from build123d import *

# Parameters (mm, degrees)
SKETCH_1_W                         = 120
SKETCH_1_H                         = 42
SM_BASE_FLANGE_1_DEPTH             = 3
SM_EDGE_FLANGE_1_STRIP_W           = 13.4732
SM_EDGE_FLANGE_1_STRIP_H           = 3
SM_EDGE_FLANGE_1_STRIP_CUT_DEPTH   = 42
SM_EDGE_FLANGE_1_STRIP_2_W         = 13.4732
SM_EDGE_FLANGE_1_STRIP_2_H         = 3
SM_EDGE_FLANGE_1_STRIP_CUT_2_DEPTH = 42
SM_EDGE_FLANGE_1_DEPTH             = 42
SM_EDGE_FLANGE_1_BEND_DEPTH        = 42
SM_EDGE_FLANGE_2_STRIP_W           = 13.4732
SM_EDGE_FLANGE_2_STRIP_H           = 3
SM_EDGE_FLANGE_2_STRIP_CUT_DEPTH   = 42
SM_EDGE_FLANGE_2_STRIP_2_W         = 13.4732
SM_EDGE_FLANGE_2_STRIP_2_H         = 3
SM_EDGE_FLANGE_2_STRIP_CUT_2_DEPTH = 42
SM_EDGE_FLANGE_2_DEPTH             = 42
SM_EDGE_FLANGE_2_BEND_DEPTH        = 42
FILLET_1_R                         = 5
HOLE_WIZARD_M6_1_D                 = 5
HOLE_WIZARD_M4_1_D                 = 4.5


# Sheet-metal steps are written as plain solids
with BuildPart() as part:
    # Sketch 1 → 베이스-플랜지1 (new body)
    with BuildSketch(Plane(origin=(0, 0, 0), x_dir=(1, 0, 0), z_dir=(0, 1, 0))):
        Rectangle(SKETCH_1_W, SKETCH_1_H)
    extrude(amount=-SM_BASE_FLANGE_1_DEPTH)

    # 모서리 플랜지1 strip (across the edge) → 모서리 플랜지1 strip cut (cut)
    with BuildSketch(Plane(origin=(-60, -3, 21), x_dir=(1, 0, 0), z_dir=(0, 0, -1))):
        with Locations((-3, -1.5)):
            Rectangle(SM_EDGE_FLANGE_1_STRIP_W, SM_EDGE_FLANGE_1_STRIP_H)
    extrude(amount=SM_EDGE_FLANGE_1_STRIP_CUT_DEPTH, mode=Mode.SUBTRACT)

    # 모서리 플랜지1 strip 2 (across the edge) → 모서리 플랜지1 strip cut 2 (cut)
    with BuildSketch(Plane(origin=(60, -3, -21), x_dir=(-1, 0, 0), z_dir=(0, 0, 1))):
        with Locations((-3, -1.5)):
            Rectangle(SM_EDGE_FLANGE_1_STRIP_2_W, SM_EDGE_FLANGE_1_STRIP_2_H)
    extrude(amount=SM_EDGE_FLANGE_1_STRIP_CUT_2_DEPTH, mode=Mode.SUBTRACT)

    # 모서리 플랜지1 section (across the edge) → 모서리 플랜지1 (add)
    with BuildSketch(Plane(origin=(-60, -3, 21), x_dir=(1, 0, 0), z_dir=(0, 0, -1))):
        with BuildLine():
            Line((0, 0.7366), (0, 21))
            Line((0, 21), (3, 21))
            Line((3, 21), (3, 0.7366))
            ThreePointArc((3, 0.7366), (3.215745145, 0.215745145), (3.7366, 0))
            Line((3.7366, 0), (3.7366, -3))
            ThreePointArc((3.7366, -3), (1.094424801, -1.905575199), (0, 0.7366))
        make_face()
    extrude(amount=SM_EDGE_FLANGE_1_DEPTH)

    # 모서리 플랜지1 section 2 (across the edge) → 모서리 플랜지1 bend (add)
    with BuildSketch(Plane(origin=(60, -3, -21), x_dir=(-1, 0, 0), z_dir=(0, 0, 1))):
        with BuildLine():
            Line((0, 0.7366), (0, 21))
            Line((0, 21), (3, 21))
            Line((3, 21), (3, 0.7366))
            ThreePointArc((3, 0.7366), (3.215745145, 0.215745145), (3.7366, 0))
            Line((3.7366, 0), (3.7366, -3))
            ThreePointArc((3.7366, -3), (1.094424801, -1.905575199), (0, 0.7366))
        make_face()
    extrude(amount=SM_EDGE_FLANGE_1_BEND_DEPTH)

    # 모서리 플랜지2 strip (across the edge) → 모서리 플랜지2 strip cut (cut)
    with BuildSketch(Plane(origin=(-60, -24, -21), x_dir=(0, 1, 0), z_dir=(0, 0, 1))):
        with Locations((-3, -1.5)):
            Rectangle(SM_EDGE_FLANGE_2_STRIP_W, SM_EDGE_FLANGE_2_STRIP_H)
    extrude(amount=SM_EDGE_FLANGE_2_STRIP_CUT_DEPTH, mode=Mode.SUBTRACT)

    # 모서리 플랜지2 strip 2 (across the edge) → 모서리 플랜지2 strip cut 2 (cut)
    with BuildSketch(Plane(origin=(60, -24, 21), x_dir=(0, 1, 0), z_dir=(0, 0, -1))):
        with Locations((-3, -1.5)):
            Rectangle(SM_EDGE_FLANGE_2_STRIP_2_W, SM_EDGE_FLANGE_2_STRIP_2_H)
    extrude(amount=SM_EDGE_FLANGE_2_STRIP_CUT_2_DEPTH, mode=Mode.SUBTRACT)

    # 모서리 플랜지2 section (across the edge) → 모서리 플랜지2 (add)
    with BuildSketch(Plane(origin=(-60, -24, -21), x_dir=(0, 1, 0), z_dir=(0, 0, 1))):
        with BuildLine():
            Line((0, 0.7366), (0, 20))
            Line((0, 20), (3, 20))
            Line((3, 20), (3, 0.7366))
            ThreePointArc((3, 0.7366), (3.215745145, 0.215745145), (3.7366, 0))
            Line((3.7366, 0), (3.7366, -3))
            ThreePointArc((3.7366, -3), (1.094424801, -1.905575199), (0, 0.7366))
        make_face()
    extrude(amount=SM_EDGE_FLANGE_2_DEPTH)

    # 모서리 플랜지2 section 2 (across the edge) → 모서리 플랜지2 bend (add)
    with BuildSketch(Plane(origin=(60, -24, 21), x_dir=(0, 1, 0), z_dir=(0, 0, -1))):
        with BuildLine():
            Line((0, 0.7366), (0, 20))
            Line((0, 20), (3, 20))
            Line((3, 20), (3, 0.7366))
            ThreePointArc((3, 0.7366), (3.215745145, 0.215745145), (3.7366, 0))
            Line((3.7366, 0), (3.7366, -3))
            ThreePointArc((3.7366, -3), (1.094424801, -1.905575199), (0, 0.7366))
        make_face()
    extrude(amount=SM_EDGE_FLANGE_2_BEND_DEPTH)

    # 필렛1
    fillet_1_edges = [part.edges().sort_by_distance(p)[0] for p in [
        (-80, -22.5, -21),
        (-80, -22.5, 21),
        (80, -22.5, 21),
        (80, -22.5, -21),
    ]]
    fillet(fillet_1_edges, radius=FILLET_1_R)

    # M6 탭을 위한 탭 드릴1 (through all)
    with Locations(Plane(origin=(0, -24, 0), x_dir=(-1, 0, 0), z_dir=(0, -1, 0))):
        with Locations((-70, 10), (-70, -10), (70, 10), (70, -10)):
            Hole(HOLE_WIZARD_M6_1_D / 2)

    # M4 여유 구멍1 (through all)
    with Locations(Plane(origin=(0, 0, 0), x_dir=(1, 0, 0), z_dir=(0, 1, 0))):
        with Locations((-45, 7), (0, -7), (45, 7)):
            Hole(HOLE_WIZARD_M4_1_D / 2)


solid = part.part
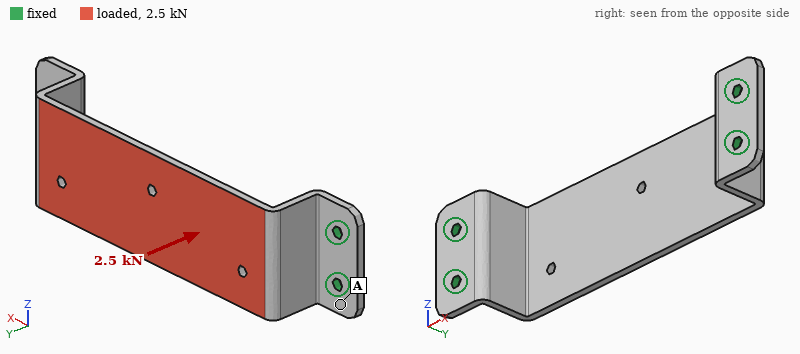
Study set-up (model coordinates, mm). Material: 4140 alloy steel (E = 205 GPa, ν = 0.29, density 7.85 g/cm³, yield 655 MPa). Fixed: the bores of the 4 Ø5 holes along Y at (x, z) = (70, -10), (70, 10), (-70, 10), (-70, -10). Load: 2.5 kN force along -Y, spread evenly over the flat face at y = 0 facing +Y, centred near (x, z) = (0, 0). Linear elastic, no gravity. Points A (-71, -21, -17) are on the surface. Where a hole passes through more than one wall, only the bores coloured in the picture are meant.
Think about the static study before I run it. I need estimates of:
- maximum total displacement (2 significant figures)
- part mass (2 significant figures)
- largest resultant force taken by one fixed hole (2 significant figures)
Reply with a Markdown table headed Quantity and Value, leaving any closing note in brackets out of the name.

| Quantity | Value |
|---|---|
| maximum total displacement | 0.74 mm |
| part mass | 190 g |
| largest resultant force taken by one fixed hole | 1.0 kN |
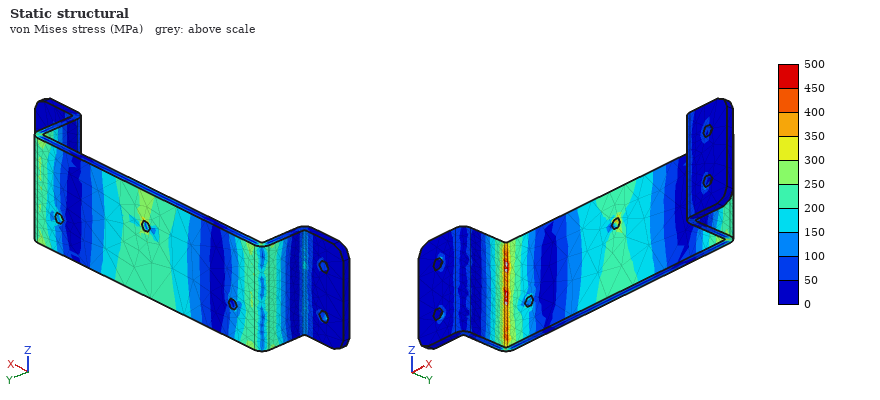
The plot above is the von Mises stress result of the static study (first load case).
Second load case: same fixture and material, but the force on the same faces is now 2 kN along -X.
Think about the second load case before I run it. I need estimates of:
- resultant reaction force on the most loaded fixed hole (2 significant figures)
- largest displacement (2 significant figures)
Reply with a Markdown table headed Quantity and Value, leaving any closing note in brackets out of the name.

| Quantity | Value |
|---|---|
| resultant reaction force on the most loaded fixed hole | 520 N |
| largest displacement | 0.21 mm |
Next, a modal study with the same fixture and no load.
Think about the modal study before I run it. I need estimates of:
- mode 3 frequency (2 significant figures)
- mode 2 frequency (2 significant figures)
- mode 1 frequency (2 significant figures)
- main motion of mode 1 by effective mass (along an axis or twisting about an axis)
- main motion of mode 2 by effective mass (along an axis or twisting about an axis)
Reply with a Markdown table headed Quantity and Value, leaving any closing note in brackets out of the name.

| Quantity | Value |
|---|---|
| mode 3 frequency | 2100 Hz |
| mode 2 frequency | 1300 Hz |
| mode 1 frequency | 1000 Hz |
| main motion of mode 1 by effective mass | along Y |
| main motion of mode 2 by effective mass | along X |
